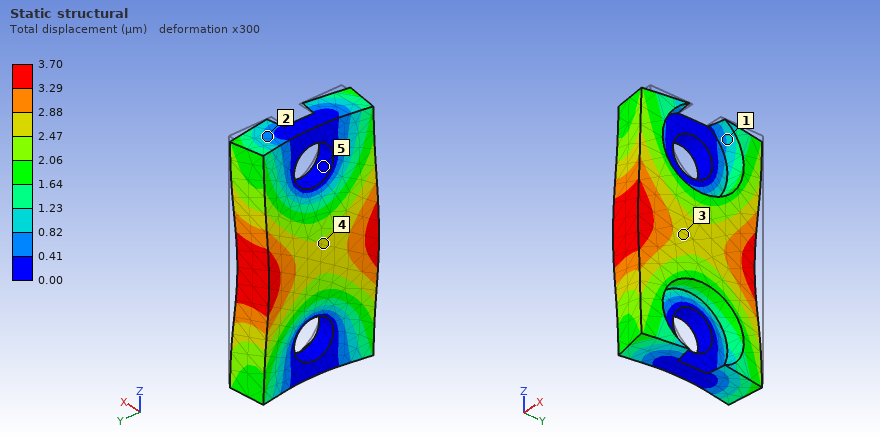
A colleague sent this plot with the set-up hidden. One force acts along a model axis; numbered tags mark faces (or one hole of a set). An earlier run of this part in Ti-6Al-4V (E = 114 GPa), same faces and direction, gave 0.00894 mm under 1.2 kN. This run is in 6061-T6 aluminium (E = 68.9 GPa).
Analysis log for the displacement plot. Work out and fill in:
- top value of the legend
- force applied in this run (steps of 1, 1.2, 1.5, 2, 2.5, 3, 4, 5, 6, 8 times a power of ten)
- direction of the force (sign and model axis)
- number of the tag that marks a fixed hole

3.70 µm
300 N
-X
5
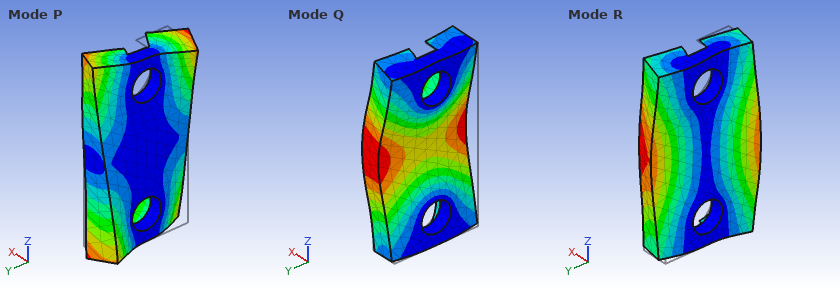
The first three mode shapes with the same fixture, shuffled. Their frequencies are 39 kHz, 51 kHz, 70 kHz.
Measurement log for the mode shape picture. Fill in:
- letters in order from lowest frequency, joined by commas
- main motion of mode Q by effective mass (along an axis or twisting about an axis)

R, Q, P
along X
